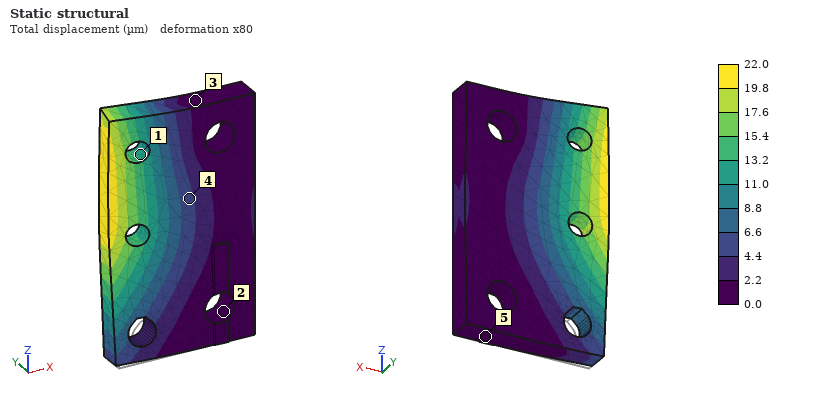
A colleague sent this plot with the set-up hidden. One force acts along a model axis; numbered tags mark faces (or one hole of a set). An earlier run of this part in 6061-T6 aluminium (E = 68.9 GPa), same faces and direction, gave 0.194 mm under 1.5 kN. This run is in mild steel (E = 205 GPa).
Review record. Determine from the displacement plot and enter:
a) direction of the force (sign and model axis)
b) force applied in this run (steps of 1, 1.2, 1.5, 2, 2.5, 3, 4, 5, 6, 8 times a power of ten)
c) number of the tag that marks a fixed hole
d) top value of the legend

+Y
500 N
2
22.0 µm
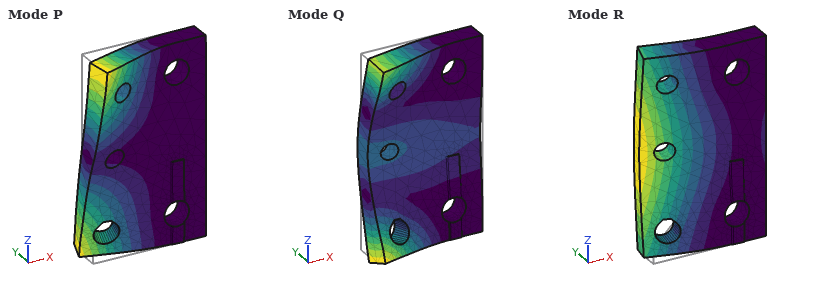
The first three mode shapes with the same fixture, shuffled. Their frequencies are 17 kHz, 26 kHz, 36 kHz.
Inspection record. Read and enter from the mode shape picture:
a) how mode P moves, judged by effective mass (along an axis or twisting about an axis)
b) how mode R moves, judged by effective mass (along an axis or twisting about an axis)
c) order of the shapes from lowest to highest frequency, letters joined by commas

twisting about X
along Y
R, P, Q
